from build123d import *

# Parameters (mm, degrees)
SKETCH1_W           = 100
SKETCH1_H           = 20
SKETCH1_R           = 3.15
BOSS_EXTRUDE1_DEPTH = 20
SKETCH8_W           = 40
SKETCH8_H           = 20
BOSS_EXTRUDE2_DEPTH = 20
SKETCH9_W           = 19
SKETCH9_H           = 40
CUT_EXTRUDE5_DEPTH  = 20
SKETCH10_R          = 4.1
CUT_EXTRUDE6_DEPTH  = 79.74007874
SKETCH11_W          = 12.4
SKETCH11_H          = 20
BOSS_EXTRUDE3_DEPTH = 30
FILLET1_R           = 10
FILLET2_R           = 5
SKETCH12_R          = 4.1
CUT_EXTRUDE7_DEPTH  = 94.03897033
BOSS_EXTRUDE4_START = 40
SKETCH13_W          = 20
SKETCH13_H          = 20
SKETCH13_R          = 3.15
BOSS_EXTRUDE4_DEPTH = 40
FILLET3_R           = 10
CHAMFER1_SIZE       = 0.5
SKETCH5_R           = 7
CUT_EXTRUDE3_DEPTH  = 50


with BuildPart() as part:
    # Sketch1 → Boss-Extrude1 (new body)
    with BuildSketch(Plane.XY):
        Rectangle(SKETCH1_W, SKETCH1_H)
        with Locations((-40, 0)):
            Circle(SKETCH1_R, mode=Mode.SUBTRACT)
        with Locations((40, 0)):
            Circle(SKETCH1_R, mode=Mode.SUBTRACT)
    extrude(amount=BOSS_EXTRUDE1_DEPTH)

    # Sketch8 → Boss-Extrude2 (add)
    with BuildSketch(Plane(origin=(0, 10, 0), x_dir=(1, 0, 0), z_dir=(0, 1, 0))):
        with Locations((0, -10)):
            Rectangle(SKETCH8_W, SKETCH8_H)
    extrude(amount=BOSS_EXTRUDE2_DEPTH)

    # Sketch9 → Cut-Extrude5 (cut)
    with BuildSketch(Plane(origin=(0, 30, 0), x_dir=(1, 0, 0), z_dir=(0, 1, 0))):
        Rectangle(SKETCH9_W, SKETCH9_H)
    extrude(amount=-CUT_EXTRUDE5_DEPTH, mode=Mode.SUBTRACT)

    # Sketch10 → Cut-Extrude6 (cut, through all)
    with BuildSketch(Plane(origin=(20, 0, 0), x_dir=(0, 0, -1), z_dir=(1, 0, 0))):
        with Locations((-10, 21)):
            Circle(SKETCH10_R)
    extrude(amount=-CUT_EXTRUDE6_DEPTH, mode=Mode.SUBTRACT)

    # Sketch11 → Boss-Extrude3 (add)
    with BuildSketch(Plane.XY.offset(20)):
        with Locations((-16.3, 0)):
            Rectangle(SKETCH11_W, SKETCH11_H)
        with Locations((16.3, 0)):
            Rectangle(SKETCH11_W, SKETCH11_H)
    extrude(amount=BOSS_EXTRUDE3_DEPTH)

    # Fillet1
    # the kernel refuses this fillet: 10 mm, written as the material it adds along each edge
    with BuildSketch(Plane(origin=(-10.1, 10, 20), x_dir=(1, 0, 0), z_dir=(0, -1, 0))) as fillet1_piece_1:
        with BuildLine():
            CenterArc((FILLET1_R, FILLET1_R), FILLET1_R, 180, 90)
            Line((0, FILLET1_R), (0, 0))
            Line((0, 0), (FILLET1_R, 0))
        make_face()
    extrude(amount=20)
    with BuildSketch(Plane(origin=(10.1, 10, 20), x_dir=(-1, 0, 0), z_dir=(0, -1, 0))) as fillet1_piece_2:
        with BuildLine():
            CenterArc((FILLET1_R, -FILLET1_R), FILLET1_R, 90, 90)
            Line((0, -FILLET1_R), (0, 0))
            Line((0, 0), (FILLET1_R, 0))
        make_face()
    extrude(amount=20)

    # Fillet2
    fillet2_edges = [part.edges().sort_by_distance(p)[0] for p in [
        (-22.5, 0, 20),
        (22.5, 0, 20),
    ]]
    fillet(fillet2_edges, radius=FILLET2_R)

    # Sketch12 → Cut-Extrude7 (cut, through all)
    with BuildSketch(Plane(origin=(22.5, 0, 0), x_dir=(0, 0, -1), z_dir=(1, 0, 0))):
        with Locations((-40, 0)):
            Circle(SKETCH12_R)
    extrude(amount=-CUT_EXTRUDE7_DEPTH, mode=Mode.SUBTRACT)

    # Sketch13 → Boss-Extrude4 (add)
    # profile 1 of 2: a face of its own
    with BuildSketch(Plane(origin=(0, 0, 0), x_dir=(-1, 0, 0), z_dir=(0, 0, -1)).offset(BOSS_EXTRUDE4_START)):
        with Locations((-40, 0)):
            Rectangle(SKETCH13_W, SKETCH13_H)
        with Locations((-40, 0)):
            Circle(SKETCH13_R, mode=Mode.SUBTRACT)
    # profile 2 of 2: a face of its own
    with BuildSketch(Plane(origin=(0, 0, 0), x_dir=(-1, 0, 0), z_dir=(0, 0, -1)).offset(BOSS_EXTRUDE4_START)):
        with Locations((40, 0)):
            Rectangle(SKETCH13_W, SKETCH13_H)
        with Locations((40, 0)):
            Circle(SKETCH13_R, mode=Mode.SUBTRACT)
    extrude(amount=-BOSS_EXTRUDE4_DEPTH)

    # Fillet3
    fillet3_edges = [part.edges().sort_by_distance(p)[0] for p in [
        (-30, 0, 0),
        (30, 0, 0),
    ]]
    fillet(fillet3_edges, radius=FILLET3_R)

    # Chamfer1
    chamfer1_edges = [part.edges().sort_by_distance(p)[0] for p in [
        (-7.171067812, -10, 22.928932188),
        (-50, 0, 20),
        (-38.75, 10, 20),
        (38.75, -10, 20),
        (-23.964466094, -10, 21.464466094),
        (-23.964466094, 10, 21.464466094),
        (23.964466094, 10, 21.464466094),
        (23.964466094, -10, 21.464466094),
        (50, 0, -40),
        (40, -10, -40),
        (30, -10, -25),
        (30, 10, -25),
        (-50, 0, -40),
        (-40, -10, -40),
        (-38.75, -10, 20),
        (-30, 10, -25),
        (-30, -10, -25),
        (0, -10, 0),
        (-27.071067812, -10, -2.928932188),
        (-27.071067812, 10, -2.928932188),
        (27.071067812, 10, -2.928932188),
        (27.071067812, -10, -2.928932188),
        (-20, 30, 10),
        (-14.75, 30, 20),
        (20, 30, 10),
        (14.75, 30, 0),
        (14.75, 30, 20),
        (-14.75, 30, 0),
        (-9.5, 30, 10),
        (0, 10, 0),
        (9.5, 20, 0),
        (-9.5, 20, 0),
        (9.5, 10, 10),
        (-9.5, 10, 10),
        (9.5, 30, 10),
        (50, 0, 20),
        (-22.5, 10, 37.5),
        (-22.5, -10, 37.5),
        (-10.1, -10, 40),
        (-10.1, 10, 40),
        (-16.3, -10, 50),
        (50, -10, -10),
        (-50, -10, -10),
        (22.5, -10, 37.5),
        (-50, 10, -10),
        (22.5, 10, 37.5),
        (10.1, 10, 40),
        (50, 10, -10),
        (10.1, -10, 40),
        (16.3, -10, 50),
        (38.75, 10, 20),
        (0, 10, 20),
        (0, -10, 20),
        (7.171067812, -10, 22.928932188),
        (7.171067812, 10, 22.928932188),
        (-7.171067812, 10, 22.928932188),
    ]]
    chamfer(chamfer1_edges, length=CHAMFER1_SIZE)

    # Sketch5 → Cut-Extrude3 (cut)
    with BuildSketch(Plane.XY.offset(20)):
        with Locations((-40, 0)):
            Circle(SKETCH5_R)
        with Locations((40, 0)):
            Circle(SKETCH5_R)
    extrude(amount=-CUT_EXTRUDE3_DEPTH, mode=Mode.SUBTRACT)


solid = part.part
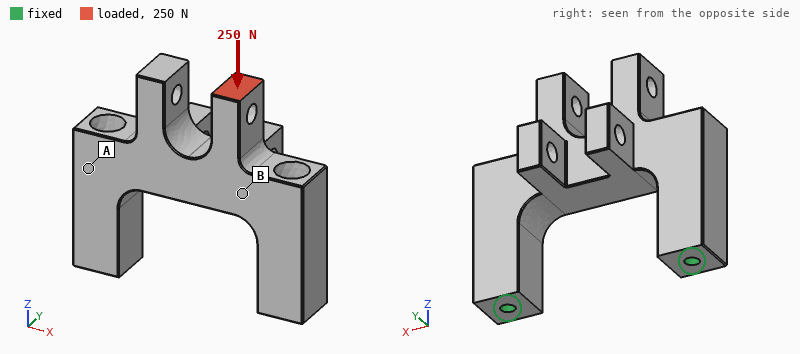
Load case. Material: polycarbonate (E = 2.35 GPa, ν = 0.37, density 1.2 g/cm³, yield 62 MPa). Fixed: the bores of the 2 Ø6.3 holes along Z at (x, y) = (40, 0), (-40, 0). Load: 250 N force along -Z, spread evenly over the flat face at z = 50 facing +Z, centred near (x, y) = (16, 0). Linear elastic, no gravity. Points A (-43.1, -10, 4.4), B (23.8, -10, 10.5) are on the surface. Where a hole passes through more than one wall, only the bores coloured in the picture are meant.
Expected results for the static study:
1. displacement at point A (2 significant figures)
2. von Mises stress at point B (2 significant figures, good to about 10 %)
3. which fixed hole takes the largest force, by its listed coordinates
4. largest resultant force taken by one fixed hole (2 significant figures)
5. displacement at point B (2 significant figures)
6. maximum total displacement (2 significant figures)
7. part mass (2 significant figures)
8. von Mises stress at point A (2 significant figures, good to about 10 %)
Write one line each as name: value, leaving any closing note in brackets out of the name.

displacement at point A: 10 µm
von Mises stress at point B: 0.92 MPa
which fixed hole takes the largest force, by its listed coordinates: (40, 0)
largest resultant force taken by one fixed hole: 180 N
displacement at point B: 31 µm
maximum total displacement: 58 µm
part mass: 94 g
von Mises stress at point A: 0.36 MPa
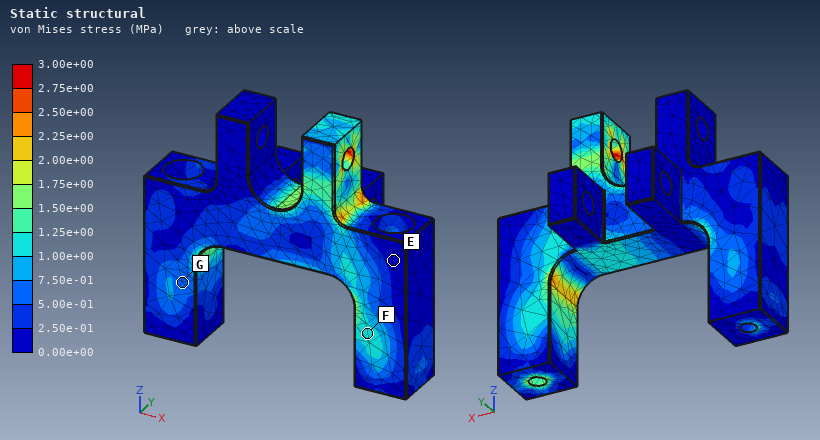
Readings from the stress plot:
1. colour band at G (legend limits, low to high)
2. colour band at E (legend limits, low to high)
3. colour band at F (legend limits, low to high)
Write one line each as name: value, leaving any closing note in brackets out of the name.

colour band at G: 5.00e-01 to 7.50e-01 MPa
colour band at E: 0.00e+00 to 2.50e-01 MPa
colour band at F: 1.00e+00 to 1.25e+00 MPa
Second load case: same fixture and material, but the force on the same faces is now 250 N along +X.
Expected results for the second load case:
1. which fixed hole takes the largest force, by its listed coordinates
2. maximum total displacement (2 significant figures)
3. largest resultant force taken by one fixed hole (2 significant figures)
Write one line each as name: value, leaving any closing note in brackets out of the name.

which fixed hole takes the largest force, by its listed coordinates: (-40, 0)
maximum total displacement: 0.53 mm
largest resultant force taken by one fixed hole: 270 N
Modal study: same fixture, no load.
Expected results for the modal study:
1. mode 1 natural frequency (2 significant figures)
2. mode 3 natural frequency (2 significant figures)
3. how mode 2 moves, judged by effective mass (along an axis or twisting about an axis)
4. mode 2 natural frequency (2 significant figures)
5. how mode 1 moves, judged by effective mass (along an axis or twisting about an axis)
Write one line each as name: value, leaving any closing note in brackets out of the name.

mode 1 natural frequency: 410 Hz
mode 3 natural frequency: 1100 Hz
how mode 2 moves, judged by effective mass: along X
mode 2 natural frequency: 900 Hz
how mode 1 moves, judged by effective mass: along Y
